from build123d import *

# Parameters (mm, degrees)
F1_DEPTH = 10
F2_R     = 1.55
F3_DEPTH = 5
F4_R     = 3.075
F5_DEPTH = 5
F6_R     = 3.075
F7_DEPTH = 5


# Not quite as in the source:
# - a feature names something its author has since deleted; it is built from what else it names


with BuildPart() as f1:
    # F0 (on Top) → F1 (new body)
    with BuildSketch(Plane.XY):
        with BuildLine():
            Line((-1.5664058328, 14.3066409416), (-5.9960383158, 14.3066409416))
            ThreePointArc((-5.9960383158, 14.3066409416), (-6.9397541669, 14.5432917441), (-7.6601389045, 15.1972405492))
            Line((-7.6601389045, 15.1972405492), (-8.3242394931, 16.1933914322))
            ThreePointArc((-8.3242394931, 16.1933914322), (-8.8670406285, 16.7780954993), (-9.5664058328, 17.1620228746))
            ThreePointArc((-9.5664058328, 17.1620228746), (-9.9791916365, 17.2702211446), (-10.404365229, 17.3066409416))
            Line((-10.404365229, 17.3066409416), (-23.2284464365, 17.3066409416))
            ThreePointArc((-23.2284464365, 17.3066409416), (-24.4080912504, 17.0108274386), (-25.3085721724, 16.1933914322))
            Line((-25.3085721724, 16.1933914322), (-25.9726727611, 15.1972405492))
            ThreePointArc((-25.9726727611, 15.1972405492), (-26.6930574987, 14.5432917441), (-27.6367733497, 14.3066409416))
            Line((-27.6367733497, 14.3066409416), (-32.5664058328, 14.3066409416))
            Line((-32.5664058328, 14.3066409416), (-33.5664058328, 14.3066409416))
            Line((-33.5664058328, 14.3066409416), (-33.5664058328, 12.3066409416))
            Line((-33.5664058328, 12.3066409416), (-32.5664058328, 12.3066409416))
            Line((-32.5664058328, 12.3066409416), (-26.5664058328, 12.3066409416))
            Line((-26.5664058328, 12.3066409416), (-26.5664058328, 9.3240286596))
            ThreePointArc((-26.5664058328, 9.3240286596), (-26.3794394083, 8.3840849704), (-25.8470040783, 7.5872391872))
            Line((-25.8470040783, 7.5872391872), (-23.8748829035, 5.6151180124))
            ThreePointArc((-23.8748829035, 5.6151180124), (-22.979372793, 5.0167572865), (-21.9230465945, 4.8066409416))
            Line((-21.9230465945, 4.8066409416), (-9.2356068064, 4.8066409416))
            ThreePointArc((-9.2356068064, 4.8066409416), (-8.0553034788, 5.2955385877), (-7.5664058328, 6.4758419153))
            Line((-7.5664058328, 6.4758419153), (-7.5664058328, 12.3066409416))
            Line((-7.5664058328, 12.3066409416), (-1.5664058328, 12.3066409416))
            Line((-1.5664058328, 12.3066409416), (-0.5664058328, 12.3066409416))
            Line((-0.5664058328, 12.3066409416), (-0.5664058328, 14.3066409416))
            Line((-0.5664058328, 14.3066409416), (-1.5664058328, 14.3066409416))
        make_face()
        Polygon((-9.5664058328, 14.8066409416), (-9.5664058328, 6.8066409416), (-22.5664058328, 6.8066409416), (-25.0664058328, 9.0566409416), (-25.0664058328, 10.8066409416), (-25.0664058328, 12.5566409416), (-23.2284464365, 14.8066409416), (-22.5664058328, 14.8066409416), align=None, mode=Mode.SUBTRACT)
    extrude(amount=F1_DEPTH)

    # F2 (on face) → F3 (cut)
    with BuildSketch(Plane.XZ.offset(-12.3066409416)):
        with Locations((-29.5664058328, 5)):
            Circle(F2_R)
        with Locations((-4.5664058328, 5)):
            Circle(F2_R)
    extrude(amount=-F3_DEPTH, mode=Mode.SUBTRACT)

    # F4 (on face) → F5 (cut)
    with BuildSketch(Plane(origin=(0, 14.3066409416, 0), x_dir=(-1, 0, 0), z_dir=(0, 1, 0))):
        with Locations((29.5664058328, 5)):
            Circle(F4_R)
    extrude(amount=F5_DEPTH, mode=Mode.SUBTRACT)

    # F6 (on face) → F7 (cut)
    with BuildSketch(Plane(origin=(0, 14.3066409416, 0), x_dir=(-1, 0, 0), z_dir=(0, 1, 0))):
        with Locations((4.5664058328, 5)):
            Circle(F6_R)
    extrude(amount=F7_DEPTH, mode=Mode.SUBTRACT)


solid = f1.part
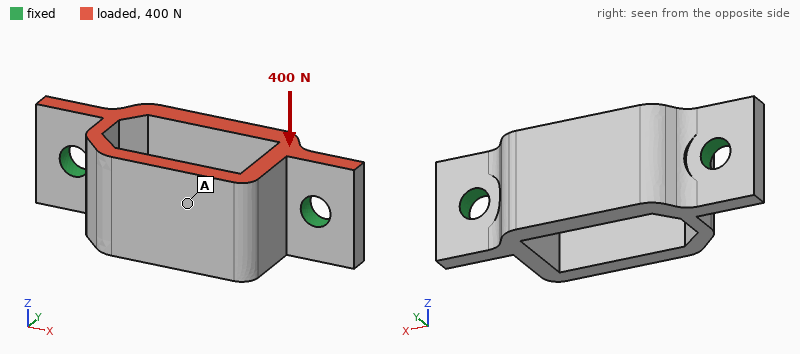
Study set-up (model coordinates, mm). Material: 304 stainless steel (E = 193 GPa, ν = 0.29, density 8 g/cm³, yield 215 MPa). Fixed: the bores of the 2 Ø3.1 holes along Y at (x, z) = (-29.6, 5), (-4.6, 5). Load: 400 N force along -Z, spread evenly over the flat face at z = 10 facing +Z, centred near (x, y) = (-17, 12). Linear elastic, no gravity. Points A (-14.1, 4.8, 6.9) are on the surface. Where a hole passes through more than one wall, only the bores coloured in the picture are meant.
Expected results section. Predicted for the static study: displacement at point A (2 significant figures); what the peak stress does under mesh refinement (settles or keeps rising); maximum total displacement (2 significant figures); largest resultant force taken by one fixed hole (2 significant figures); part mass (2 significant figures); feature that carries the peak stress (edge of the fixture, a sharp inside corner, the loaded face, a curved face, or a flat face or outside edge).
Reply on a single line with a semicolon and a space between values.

3.9 µm; keeps rising; 4.3 µm; 210 N; 11 g; edge of the fixture
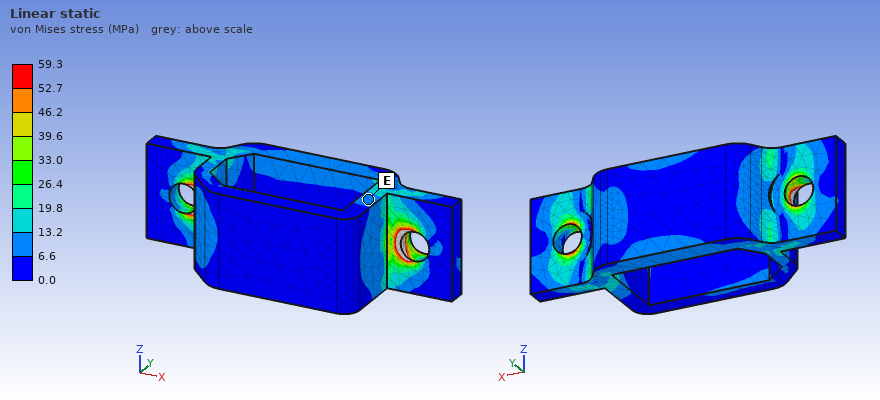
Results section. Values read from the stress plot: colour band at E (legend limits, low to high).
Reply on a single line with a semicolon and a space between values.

6.6 to 13.2 MPa
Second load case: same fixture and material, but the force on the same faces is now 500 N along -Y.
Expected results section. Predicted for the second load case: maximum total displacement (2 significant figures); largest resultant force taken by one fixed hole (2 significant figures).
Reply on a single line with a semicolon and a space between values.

14 µm; 270 N
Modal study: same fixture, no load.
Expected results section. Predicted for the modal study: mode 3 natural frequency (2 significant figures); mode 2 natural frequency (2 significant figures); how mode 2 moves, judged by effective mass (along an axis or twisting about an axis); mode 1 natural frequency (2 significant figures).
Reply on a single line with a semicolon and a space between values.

25 kHz; 16 kHz; along X; 14 kHz
